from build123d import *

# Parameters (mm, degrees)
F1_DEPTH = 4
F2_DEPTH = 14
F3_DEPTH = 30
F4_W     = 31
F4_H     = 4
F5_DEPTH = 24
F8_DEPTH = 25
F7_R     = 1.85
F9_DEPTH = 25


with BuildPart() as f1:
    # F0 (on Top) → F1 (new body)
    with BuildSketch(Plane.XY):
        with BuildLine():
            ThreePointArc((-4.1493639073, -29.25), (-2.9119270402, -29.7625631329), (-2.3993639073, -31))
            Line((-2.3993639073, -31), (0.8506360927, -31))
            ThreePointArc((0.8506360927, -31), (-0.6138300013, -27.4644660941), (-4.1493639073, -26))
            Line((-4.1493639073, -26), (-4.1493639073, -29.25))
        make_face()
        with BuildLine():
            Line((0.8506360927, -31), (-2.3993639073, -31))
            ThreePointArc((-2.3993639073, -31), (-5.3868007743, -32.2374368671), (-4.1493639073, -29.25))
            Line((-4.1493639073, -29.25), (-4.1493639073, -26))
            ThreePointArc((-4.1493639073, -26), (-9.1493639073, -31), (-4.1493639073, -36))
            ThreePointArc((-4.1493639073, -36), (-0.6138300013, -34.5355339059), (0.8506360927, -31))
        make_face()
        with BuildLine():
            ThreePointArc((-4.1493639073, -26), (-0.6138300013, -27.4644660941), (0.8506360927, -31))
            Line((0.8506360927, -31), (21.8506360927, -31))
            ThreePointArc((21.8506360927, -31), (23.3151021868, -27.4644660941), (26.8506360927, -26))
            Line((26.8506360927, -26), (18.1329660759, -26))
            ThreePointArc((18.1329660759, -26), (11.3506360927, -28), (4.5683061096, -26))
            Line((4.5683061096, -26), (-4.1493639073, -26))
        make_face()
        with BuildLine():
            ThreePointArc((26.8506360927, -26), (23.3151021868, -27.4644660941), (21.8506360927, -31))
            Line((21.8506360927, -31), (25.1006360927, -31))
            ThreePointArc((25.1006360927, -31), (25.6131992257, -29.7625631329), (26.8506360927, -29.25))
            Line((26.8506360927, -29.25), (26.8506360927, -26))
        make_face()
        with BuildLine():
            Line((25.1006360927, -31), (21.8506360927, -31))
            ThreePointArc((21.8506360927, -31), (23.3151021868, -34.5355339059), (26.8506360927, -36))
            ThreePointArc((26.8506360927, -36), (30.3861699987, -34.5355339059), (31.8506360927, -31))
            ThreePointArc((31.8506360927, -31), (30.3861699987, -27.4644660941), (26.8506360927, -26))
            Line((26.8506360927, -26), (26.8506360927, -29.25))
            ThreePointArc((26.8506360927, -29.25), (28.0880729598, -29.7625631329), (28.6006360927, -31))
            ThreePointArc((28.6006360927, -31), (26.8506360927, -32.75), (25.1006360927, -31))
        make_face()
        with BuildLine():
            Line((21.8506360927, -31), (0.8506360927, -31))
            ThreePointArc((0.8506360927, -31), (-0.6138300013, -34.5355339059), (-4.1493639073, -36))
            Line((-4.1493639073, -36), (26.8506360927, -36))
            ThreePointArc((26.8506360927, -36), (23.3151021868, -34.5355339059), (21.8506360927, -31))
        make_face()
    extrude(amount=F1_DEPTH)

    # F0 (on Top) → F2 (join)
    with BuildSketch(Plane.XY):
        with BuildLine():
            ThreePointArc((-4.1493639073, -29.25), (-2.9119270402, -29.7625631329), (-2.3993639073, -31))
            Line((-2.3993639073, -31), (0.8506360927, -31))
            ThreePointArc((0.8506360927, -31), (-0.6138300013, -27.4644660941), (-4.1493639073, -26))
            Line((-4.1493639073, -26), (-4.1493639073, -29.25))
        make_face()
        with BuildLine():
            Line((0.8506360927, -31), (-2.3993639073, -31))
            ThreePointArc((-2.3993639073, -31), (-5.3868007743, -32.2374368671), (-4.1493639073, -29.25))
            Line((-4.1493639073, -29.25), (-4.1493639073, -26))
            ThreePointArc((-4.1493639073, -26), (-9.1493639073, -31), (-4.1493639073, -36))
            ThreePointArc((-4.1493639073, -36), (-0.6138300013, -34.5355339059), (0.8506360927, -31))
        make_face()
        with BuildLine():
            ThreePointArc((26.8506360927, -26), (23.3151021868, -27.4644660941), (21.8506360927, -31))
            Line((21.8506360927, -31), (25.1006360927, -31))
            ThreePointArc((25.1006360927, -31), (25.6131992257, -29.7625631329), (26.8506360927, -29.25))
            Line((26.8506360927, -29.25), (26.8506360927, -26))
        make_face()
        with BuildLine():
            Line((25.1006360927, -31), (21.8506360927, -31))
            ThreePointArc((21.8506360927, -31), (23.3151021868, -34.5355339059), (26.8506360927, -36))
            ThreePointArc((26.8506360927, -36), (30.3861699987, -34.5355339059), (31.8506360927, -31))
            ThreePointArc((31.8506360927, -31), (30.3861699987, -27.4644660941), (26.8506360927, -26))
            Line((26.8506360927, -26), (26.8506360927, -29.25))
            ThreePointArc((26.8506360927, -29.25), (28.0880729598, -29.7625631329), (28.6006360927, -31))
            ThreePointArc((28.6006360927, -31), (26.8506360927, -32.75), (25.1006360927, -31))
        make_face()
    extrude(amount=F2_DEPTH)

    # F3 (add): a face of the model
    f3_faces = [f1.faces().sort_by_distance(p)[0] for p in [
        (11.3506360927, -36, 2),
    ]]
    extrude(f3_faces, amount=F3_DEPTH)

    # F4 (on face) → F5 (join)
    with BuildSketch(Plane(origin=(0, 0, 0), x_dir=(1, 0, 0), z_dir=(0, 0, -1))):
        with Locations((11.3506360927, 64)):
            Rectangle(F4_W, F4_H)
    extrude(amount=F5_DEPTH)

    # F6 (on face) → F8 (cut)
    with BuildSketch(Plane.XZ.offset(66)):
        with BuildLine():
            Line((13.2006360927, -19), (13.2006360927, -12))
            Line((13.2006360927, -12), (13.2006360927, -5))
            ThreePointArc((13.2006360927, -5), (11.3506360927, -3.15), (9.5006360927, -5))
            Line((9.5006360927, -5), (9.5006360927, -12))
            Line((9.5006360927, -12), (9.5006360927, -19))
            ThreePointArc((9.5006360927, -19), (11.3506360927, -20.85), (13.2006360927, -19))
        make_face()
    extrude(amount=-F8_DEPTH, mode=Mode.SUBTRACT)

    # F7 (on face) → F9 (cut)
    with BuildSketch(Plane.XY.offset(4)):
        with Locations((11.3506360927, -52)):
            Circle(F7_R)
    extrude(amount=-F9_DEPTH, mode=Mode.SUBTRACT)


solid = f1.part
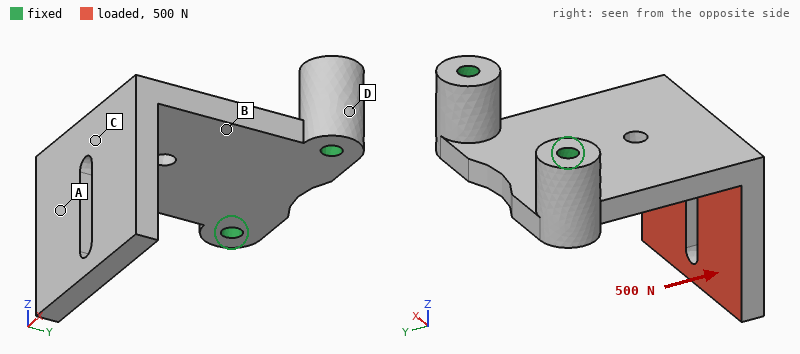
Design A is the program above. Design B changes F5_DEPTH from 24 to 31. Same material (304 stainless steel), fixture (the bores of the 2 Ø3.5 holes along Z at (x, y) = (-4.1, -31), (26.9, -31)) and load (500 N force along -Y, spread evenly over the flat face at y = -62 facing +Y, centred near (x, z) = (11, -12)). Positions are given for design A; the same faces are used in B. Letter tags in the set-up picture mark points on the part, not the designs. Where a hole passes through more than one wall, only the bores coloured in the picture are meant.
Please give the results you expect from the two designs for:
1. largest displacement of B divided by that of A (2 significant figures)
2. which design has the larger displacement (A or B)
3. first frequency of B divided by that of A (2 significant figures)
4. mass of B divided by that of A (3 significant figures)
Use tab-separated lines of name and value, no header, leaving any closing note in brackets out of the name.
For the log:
largest displacement of B divided by that of A	1.6
which design has the larger displacement	B
first frequency of B divided by that of A	0.81
mass of B divided by that of A	1.09
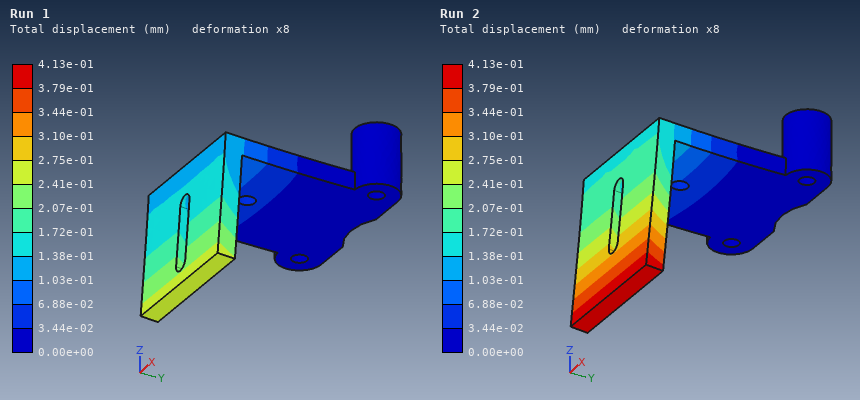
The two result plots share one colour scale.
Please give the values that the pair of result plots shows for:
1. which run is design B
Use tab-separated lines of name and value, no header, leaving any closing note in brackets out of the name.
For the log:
which run is design B	Run 2
